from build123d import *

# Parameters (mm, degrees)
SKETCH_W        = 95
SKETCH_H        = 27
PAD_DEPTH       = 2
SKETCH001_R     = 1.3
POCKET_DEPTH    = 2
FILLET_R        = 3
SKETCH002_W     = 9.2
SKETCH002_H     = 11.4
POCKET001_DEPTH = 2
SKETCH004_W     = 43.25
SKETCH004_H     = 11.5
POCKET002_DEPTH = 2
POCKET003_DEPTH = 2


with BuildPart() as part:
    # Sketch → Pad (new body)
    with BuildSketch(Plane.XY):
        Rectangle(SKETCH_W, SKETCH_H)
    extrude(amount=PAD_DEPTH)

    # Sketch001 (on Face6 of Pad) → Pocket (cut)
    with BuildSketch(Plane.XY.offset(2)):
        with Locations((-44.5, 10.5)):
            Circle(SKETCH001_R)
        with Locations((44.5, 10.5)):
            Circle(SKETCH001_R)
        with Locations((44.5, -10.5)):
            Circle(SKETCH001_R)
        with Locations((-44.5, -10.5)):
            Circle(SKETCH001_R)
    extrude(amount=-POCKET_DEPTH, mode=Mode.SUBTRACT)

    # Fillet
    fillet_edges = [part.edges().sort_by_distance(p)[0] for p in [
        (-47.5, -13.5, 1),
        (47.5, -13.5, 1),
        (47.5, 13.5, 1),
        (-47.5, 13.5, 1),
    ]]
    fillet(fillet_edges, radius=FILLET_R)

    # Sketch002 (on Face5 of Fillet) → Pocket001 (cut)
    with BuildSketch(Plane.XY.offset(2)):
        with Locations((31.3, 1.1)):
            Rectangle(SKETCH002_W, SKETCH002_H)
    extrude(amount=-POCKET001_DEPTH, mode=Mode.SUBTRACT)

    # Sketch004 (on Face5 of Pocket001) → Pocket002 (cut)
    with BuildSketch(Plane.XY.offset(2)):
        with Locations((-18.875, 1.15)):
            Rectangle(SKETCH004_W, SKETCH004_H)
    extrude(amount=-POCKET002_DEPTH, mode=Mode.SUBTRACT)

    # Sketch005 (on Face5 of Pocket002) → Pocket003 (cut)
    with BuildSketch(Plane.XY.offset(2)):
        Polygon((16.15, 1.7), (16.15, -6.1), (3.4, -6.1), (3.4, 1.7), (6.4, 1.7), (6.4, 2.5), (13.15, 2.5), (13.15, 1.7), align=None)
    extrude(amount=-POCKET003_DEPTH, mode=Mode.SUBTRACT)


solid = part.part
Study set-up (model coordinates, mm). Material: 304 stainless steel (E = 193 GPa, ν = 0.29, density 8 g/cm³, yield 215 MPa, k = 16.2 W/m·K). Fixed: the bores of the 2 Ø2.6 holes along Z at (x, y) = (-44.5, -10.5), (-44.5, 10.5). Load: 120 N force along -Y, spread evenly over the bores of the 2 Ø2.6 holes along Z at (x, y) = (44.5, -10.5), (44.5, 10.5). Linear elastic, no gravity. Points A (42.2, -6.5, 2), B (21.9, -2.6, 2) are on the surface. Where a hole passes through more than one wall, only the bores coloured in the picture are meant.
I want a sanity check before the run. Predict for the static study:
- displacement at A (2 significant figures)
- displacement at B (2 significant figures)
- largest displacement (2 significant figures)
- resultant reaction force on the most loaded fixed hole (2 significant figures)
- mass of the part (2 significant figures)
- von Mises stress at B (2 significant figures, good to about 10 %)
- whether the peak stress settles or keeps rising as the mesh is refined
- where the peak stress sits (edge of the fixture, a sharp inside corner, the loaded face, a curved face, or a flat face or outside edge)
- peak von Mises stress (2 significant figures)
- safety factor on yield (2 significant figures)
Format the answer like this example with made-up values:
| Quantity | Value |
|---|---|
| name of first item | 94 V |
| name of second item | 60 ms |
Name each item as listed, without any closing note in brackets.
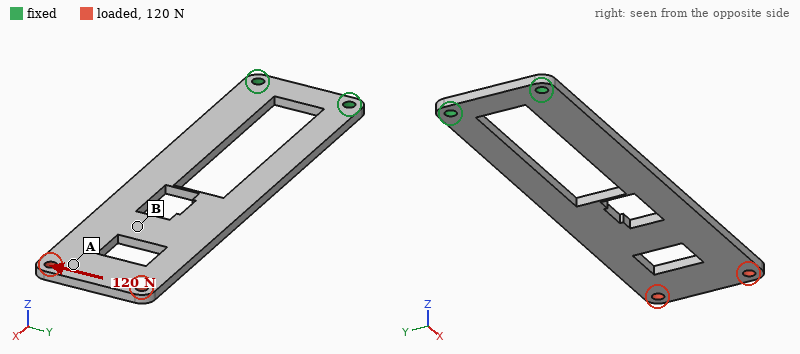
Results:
| Quantity | Value |
|---|---|
| displacement at A | 0.12 mm |
| displacement at B | 0.10 mm |
| largest displacement | 0.13 mm |
| resultant reaction force on the most loaded fixed hole | 450 N |
| mass of the part | 29 g |
| von Mises stress at B | 29 MPa |
| whether the peak stress settles or keeps rising as the mesh is refined | settles |
| where the peak stress sits | a flat face or outside edge |
| peak von Mises stress | 180 MPa |
| safety factor on yield | 1.2 |
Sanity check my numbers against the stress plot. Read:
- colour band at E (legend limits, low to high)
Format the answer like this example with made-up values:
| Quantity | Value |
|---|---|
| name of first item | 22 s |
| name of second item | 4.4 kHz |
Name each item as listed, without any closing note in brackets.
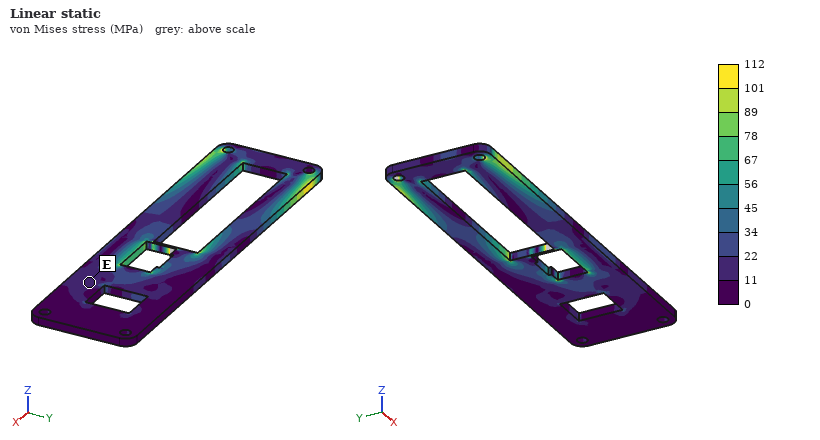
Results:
| Quantity | Value |
|---|---|
| colour band at E | 11 to 22 MPa |
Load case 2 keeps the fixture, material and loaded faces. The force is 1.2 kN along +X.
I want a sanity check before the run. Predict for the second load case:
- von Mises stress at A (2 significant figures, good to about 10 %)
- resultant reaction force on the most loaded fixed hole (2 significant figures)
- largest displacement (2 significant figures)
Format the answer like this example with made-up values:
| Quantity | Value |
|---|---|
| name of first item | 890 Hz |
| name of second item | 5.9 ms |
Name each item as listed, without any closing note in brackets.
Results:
| Quantity | Value |
|---|---|
| von Mises stress at A | 25 MPa |
| resultant reaction force on the most loaded fixed hole | 610 N |
| largest displacement | 21 µm |
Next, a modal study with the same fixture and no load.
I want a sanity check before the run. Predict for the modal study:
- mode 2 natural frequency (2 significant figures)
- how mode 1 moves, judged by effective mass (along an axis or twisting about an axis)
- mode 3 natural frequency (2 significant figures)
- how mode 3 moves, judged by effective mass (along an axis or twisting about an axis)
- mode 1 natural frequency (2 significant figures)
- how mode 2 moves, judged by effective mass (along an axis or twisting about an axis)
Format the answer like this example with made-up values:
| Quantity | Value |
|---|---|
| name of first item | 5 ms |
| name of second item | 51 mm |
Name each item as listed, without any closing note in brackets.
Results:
| Quantity | Value |
|---|---|
| mode 2 natural frequency | 990 Hz |
| how mode 1 moves, judged by effective mass | along Z |
| mode 3 natural frequency | 1100 Hz |
| how mode 3 moves, judged by effective mass | along Z |
| mode 1 natural frequency | 160 Hz |
| how mode 2 moves, judged by effective mass | twisting about X |
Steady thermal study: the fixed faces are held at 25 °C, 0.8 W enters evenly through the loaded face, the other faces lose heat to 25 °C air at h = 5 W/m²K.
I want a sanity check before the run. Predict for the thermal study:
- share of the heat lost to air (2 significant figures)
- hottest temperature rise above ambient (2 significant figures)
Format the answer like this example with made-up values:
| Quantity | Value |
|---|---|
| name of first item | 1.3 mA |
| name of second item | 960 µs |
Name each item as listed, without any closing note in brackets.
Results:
| Quantity | Value |
|---|---|
| share of the heat lost to air | 73 % |
| hottest temperature rise above ambient | 62 K |
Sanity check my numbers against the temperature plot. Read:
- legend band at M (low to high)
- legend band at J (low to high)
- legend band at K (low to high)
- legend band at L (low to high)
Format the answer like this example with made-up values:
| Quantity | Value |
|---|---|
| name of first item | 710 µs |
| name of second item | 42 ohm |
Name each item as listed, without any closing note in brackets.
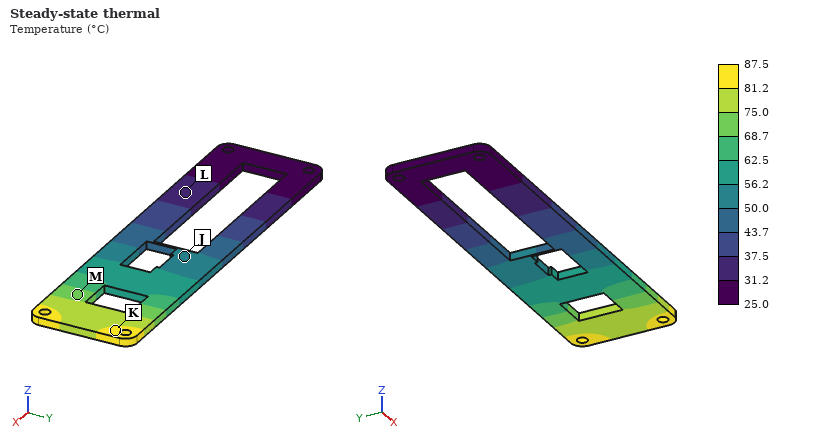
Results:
| Quantity | Value |
|---|---|
| legend band at M | 68.7 to 75.0 °C |
| legend band at J | 50.0 to 56.2 °C |
| legend band at K | 81.2 to 87.5 °C |
| legend band at L | 31.2 to 37.5 °C |
